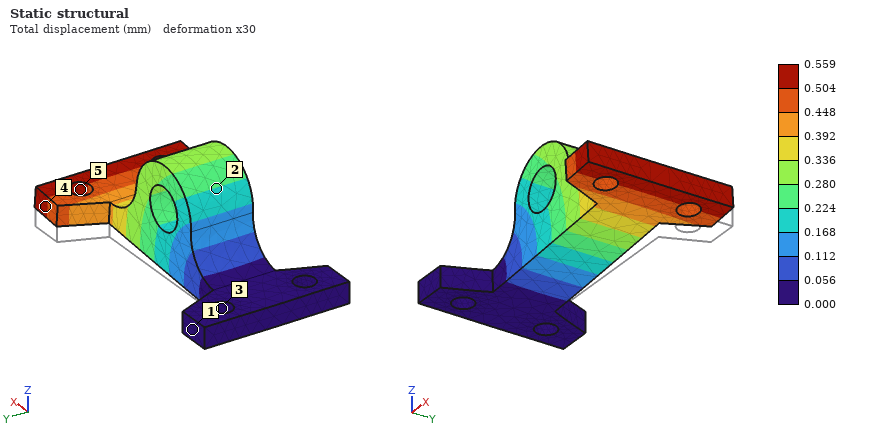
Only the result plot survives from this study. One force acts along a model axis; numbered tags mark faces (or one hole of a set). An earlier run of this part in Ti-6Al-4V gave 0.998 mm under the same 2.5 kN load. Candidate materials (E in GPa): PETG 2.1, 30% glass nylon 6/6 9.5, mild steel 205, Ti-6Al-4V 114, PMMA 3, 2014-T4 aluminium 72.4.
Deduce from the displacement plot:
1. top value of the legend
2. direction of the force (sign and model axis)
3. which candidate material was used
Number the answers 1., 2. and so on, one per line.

1. 0.559 mm
2. +Z
3. mild steel
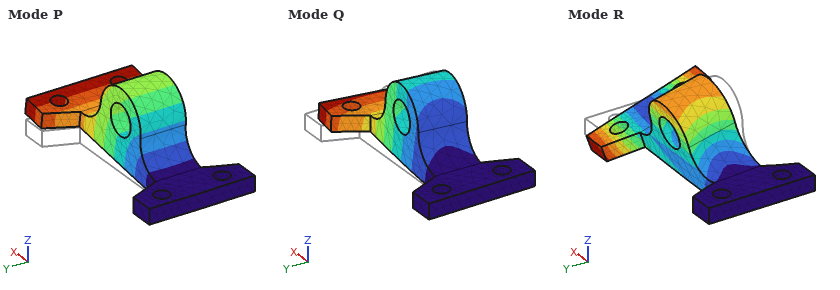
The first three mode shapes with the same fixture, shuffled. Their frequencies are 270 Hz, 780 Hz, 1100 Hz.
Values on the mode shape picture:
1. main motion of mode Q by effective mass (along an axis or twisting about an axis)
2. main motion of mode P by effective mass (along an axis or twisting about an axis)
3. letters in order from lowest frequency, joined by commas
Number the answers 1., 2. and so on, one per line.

1. along Y
2. along Z
3. P, Q, R
